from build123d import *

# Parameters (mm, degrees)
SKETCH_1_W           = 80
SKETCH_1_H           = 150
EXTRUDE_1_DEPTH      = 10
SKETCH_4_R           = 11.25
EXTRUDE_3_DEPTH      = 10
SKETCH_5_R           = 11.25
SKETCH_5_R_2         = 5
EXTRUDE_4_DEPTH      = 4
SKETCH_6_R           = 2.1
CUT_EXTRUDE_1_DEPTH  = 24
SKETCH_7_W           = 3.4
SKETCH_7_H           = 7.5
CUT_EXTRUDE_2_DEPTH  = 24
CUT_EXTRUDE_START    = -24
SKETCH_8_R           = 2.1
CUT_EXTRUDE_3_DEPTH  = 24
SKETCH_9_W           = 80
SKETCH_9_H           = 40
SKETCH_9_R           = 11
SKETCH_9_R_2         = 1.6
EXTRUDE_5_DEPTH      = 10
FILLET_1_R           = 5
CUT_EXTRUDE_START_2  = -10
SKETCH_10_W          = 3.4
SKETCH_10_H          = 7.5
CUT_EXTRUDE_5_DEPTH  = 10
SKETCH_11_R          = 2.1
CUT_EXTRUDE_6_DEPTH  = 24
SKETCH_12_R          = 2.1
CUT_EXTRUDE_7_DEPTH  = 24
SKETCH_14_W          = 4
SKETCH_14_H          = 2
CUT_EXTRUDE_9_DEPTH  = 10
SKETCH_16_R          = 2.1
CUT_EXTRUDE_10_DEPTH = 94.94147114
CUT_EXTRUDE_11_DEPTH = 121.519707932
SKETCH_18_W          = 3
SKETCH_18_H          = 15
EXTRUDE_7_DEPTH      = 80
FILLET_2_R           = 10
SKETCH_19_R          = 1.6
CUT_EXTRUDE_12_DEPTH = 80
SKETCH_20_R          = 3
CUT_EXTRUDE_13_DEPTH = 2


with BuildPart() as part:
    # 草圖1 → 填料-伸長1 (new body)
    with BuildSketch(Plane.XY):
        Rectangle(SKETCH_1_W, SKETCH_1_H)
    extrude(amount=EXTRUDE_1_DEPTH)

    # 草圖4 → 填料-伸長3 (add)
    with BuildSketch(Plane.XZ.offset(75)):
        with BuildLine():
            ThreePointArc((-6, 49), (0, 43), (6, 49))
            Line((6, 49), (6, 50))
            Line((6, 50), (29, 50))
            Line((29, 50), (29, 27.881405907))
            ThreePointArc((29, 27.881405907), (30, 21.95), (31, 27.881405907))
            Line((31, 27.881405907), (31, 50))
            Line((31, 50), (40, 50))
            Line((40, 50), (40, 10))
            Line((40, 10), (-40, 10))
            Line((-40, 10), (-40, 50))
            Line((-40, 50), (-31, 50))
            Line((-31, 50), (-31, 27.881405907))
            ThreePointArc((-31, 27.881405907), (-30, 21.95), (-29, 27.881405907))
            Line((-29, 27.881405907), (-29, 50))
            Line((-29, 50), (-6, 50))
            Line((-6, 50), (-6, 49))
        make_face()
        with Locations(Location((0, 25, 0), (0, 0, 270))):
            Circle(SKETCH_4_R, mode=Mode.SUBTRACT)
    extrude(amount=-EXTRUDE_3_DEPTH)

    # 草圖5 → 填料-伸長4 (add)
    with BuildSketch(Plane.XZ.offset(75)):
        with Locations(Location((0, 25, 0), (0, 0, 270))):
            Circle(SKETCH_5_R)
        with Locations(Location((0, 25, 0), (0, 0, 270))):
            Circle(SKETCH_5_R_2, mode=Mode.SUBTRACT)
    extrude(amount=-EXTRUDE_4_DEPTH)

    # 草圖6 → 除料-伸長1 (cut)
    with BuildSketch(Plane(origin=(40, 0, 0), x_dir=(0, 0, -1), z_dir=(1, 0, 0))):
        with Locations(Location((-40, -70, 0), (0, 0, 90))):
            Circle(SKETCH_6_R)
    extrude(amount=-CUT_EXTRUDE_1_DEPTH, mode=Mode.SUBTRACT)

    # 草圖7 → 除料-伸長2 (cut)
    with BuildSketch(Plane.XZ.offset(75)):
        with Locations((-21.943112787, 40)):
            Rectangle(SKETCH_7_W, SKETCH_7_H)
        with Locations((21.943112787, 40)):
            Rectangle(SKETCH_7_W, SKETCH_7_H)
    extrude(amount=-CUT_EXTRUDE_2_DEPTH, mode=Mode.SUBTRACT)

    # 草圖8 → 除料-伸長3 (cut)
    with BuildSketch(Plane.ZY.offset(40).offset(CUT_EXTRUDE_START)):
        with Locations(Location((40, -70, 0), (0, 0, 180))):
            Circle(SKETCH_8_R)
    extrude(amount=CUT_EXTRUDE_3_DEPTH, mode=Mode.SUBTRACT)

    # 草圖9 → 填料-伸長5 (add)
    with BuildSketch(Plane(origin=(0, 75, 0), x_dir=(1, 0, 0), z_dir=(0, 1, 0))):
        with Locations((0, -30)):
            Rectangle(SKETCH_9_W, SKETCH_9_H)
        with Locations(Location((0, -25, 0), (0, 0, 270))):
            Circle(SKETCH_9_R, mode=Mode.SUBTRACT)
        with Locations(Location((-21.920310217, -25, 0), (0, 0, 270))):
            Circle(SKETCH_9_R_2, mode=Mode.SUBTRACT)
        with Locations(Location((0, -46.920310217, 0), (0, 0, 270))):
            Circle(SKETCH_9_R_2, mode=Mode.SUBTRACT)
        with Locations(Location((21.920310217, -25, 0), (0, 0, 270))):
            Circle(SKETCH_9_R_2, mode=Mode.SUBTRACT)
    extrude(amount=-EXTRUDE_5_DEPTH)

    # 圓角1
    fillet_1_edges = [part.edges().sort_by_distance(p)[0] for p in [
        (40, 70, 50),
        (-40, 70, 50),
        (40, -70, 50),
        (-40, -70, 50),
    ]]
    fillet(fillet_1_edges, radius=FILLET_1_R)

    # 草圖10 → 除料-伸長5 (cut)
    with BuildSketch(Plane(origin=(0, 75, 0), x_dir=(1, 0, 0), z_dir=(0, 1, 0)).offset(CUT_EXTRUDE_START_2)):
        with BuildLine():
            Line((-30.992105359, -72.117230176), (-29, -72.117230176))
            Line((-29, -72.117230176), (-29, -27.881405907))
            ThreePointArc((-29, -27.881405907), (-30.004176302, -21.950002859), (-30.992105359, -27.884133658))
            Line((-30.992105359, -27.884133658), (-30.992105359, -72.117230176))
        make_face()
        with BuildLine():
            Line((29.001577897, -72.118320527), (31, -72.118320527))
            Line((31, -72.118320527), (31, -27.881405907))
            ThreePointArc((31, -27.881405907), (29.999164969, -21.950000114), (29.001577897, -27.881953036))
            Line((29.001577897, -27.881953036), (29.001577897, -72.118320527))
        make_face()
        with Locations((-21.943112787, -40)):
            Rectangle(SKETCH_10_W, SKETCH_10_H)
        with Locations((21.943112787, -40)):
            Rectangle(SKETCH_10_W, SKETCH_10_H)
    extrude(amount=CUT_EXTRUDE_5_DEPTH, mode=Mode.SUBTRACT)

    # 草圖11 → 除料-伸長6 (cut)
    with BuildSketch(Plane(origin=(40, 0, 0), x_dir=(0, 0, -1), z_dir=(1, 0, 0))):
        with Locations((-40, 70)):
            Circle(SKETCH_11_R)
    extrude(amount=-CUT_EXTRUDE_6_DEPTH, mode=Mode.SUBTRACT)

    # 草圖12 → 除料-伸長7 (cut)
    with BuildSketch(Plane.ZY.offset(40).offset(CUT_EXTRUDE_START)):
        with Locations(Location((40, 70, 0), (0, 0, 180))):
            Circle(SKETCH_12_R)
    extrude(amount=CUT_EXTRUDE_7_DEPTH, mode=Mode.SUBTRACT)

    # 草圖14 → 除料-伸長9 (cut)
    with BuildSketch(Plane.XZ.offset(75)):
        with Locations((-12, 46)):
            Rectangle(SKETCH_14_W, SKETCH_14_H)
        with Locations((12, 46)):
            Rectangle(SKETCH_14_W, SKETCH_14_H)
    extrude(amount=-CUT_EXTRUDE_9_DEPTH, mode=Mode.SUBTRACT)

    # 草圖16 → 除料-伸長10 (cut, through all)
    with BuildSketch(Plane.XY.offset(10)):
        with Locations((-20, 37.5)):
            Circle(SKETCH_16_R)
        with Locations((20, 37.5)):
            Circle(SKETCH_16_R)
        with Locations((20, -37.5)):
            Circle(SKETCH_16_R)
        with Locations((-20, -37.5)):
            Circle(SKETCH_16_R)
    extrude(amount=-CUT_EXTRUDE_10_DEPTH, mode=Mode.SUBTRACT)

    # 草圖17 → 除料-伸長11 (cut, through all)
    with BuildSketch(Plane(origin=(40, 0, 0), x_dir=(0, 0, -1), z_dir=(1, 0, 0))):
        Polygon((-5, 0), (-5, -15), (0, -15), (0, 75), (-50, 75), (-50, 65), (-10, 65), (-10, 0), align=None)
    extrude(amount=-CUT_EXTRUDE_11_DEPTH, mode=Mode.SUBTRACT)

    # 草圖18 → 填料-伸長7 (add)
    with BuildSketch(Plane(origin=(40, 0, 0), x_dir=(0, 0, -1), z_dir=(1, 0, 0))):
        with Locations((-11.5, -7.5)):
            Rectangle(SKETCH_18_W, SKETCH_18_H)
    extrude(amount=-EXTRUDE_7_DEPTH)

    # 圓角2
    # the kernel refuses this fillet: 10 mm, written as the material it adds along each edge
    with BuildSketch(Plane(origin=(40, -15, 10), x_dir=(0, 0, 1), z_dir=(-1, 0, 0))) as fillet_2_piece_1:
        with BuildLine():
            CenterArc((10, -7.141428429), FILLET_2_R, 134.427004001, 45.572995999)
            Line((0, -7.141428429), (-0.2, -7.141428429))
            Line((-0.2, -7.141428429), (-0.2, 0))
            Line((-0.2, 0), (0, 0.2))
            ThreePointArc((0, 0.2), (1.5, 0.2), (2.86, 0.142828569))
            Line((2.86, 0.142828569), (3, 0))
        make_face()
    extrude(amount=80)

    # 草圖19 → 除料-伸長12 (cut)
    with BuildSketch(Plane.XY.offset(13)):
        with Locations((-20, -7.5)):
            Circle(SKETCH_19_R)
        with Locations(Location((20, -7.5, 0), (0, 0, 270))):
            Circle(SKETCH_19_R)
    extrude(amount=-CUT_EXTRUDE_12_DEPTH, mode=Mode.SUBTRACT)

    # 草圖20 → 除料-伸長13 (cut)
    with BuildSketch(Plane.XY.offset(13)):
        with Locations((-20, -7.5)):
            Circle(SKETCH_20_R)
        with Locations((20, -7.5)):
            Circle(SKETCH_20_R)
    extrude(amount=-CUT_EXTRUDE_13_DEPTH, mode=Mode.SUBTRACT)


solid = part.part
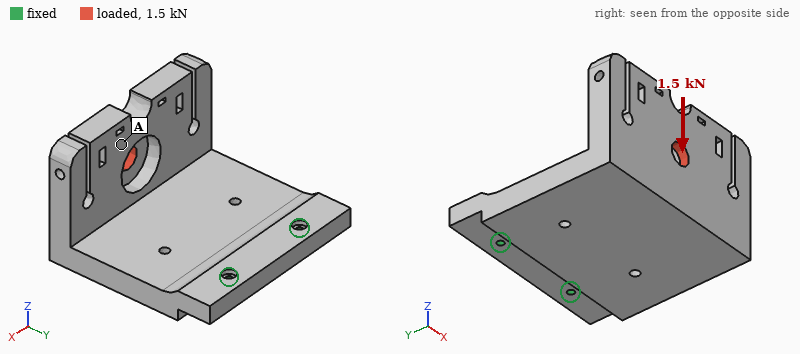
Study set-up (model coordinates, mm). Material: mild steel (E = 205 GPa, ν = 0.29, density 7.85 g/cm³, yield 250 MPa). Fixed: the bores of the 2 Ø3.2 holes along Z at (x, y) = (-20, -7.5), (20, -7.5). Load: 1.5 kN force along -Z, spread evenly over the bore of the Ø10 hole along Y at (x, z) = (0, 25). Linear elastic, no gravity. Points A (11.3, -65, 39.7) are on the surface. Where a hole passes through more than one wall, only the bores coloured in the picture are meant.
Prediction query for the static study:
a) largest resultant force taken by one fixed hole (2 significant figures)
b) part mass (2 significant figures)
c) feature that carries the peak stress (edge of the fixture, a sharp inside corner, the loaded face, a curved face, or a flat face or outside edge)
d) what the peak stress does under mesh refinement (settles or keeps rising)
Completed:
760 N
660 g
edge of the fixture
keeps rising
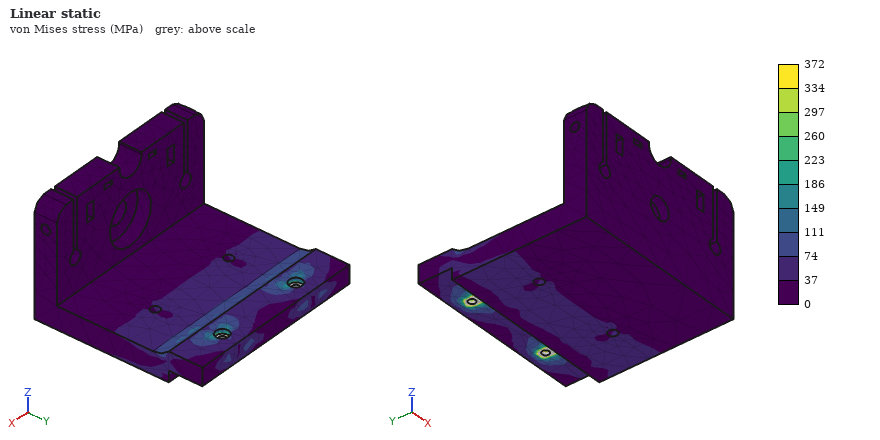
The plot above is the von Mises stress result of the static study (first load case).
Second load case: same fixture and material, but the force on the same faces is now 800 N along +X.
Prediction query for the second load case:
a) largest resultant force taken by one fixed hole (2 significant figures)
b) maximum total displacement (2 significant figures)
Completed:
1.4 kN
34 µm
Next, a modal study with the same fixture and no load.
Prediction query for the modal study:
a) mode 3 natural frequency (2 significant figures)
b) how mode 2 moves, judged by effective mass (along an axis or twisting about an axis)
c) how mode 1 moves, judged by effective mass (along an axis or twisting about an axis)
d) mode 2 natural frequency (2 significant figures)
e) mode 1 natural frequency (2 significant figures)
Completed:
2700 Hz
along X
along Z
1500 Hz
590 Hz
